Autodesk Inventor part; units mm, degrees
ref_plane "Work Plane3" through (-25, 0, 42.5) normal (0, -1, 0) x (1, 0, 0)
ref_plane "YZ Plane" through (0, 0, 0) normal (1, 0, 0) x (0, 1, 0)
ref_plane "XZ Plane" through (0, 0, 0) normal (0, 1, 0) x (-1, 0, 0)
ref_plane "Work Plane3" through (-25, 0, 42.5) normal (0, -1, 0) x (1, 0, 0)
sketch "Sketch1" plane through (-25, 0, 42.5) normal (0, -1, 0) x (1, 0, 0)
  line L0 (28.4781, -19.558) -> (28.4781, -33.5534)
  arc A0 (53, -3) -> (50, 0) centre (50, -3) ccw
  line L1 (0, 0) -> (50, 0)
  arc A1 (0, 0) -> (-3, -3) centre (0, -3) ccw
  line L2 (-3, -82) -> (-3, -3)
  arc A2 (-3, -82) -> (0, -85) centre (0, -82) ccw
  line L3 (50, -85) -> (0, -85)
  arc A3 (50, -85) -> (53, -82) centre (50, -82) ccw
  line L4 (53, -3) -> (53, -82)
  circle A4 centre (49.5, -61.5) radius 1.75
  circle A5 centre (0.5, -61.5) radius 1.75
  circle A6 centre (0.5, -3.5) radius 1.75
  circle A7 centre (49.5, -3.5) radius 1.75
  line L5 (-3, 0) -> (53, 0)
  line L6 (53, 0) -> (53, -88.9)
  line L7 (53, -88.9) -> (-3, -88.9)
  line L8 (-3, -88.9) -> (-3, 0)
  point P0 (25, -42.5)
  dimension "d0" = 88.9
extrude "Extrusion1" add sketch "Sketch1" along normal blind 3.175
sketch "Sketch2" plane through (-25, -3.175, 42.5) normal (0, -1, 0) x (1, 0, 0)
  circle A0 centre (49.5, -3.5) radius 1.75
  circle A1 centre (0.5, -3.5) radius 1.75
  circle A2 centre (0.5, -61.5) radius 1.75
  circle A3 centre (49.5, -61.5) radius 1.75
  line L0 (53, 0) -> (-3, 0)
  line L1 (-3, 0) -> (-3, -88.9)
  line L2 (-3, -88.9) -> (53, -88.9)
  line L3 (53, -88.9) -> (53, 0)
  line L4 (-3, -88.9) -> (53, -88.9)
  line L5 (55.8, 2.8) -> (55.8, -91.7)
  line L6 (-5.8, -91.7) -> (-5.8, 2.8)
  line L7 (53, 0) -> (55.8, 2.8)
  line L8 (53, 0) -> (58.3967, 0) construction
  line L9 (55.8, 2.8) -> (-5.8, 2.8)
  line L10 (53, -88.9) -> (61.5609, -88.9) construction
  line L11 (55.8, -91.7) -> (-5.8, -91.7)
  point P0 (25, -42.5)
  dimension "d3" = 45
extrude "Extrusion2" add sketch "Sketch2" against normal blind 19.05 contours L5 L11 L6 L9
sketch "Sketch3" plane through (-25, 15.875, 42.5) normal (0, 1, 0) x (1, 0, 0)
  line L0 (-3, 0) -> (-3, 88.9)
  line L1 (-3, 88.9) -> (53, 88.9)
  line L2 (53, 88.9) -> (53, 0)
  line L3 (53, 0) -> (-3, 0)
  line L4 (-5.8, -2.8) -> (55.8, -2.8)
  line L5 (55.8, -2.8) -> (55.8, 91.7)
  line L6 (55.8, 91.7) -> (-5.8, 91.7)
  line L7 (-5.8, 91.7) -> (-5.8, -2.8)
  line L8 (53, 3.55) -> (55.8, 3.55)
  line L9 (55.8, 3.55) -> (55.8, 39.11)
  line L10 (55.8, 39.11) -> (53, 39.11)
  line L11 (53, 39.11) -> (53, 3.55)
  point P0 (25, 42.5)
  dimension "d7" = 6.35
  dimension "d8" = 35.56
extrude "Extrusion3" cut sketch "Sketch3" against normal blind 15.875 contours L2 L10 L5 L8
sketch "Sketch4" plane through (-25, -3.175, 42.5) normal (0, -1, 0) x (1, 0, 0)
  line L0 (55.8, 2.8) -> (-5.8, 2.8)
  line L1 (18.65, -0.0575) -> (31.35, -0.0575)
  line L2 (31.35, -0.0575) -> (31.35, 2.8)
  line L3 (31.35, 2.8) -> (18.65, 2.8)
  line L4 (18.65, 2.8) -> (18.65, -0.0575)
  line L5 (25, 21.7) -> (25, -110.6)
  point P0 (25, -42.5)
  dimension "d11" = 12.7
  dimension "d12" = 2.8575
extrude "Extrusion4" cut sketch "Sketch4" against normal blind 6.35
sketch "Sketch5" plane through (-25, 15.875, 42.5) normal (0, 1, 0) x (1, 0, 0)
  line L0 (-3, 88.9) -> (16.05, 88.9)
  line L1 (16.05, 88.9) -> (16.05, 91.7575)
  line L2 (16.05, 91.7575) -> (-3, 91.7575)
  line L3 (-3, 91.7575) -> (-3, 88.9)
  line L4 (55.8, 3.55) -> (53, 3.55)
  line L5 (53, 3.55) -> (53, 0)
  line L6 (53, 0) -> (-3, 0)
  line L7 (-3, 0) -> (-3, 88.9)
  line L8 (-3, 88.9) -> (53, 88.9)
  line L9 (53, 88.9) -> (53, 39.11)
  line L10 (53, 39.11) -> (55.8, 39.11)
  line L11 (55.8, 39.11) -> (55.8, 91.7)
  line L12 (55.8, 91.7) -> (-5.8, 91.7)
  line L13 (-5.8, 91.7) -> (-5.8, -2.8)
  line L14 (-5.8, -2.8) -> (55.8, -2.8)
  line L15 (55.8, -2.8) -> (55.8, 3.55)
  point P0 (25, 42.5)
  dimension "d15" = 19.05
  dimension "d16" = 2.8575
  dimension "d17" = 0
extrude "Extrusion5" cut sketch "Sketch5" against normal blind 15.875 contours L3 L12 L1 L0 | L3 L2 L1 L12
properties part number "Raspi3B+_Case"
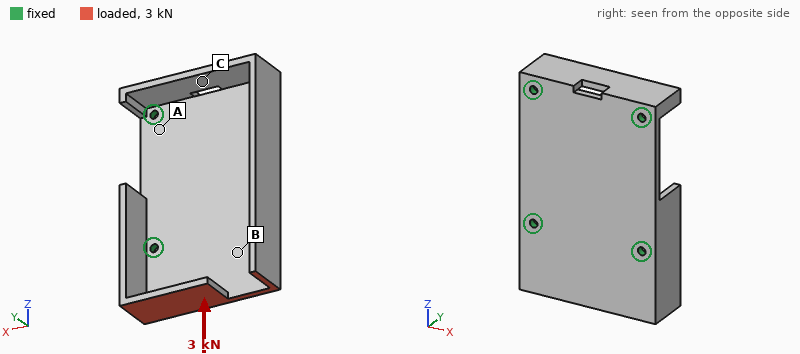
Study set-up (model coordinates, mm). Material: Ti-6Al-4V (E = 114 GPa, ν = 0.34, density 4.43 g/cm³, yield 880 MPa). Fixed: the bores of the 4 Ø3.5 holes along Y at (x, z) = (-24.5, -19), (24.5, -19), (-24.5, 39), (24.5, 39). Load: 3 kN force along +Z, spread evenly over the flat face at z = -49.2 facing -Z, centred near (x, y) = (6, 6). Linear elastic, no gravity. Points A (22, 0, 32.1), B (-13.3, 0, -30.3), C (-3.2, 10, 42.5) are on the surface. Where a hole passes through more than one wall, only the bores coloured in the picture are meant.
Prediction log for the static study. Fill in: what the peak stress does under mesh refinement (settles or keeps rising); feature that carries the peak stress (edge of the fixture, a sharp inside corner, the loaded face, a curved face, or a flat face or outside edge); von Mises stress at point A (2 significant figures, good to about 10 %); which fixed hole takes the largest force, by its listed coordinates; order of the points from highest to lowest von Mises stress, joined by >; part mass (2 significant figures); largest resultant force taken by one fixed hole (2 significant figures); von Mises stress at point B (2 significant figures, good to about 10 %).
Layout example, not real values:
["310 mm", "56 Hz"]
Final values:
["keeps rising", "edge of the fixture", "35 MPa", "(24.5, -19)", "B > A > C", "130 g", "1.5 kN", "56 MPa"]
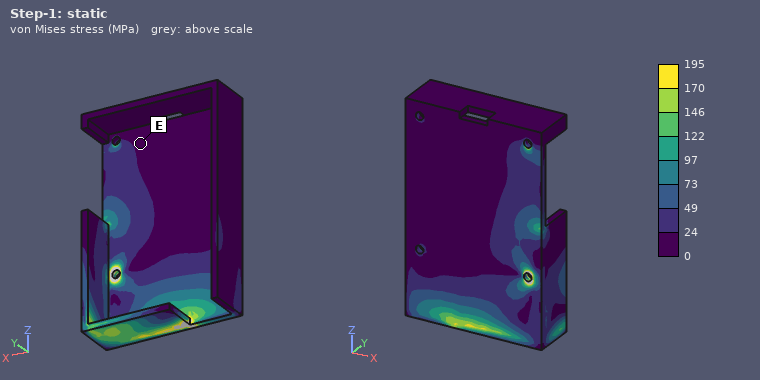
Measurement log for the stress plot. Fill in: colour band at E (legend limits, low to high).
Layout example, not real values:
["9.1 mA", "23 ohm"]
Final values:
["0 to 24 MPa"]
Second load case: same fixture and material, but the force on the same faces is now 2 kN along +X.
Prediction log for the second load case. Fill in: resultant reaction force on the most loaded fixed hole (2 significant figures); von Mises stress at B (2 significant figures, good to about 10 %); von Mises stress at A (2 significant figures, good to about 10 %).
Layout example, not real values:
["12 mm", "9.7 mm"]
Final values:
["1.6 kN", "30 MPa", "14 MPa"]
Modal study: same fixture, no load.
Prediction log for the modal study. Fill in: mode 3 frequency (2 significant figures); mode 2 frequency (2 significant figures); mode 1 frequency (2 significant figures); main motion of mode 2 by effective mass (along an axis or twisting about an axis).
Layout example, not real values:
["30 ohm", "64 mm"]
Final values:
["4700 Hz", "3900 Hz", "2600 Hz", "along Y"]
